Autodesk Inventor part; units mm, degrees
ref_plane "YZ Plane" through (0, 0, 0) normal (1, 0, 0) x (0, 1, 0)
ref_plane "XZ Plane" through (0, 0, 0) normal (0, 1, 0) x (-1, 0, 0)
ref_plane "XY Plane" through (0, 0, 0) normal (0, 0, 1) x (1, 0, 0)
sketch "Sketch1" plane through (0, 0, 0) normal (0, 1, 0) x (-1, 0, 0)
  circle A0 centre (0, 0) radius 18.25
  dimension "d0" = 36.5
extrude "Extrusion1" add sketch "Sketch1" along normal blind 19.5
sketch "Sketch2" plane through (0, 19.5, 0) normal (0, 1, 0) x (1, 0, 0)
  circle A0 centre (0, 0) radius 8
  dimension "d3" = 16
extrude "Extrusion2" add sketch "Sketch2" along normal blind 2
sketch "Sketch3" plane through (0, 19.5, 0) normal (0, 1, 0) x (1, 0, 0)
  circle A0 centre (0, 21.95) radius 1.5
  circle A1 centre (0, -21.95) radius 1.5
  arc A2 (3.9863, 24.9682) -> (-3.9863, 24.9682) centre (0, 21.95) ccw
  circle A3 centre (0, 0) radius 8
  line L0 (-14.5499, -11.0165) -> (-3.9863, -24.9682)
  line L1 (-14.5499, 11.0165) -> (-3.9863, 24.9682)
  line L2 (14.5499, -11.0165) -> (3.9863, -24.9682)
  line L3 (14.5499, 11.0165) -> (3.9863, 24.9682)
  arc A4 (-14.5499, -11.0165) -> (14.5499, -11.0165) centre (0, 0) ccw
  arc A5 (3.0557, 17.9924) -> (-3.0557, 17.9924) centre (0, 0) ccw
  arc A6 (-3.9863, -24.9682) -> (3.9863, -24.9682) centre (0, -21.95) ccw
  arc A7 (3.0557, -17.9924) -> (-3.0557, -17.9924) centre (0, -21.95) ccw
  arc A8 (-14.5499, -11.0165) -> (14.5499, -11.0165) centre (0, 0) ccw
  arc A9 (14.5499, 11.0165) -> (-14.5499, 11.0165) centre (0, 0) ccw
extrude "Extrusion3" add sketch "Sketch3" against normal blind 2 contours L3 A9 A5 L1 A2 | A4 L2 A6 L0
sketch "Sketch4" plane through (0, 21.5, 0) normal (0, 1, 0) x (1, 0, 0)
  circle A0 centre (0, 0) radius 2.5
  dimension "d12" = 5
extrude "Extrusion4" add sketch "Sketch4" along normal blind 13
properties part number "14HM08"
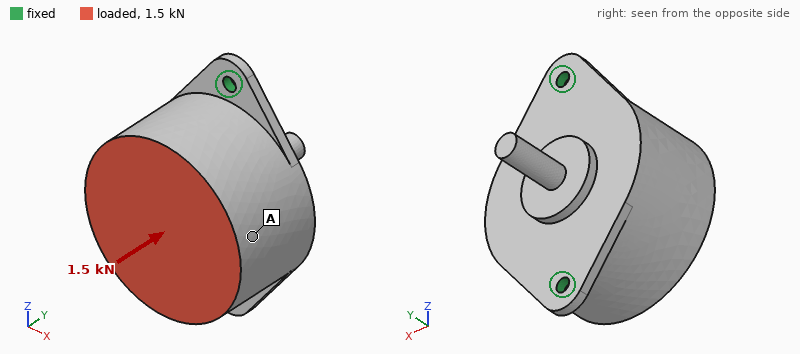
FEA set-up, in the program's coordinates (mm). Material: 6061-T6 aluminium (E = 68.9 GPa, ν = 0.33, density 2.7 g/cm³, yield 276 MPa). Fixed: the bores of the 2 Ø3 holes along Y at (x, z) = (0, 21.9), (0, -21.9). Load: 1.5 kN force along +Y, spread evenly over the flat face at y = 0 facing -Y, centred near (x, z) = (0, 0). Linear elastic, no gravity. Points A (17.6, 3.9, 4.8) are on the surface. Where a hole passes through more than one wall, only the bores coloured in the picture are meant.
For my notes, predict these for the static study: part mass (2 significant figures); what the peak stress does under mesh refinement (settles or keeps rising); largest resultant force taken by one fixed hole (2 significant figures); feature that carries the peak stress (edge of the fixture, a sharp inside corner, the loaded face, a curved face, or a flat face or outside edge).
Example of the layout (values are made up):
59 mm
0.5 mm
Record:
58 g
keeps rising
850 N
edge of the fixture
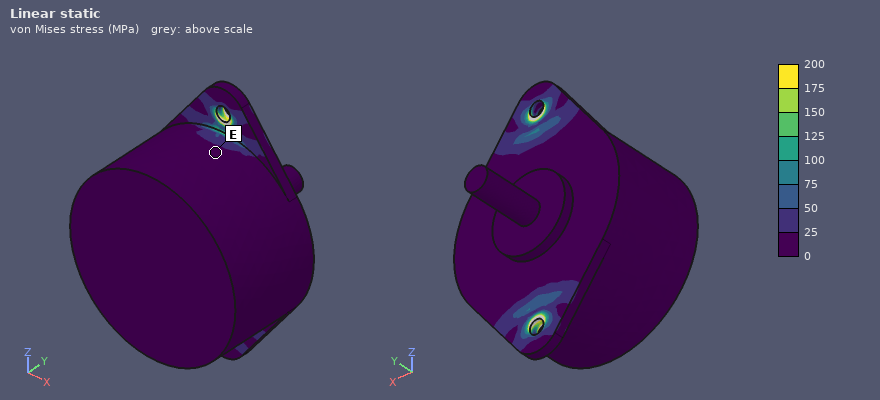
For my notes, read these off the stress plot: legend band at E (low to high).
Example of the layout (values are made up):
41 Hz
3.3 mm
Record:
0 to 25 MPa
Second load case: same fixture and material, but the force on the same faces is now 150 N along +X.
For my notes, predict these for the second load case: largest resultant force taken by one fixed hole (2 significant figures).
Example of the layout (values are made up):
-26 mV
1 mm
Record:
75 N
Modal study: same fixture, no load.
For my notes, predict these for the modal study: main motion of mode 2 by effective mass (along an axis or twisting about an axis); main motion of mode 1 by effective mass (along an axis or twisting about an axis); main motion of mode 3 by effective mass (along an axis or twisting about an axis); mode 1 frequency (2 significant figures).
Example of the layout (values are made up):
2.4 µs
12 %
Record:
along Y
along X
along Z
1200 Hz
